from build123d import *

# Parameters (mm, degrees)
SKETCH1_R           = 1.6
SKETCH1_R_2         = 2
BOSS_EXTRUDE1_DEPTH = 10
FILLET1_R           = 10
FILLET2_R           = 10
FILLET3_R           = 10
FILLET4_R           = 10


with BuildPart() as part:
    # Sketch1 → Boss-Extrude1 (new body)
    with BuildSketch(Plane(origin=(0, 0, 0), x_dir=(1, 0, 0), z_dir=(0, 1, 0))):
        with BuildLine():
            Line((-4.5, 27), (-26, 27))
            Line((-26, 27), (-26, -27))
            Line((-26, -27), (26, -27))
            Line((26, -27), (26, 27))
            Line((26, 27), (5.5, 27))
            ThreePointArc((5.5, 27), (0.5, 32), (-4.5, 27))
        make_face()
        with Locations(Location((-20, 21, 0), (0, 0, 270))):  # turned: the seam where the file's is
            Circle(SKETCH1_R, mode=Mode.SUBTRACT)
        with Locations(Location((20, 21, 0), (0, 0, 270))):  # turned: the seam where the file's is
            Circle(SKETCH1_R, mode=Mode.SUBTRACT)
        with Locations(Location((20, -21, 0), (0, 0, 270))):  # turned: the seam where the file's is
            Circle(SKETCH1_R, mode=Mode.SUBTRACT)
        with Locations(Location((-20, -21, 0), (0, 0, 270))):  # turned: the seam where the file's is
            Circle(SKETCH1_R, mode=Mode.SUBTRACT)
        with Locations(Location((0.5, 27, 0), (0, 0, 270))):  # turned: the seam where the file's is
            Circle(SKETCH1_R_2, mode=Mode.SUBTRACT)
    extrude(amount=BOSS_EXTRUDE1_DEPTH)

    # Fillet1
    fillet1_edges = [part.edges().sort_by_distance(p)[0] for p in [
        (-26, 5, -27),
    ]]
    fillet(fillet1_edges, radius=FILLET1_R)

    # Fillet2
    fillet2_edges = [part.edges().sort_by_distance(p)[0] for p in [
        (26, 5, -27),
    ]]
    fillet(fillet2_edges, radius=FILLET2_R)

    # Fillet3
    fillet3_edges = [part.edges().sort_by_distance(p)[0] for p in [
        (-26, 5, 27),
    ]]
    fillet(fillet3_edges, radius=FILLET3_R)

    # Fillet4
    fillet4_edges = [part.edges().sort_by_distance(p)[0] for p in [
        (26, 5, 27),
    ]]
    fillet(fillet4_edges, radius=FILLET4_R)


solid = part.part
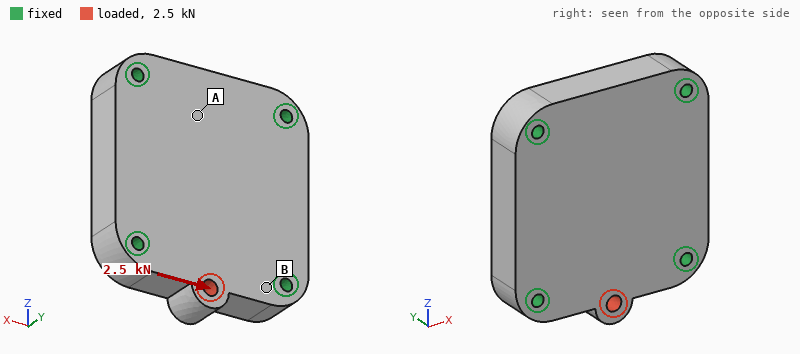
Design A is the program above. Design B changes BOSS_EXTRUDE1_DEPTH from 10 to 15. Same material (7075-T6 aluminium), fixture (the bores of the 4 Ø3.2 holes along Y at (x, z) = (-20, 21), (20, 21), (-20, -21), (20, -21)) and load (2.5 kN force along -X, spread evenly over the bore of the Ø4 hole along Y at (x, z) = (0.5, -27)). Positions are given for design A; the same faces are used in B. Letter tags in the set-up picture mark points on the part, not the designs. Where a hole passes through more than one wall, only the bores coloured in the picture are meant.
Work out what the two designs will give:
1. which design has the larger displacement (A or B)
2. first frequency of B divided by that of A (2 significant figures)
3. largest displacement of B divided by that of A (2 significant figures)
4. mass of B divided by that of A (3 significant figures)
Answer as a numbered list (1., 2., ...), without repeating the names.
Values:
1. A
2. 1.2
3. 0.66
4. 1.50
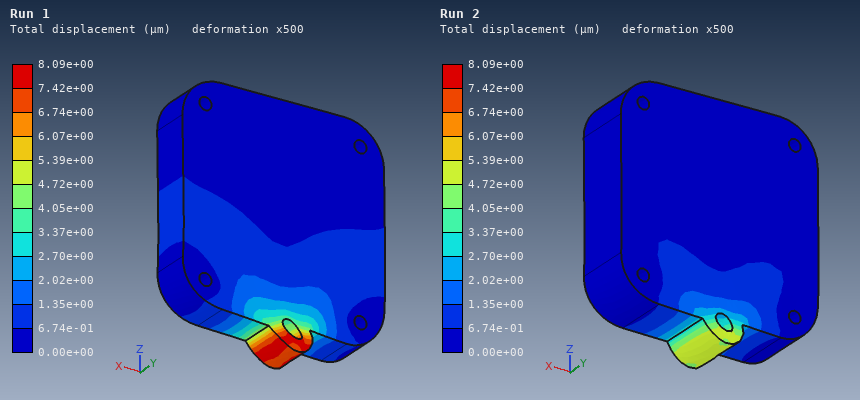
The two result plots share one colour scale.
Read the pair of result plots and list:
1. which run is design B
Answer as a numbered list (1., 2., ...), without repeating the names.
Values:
1. Run 2
